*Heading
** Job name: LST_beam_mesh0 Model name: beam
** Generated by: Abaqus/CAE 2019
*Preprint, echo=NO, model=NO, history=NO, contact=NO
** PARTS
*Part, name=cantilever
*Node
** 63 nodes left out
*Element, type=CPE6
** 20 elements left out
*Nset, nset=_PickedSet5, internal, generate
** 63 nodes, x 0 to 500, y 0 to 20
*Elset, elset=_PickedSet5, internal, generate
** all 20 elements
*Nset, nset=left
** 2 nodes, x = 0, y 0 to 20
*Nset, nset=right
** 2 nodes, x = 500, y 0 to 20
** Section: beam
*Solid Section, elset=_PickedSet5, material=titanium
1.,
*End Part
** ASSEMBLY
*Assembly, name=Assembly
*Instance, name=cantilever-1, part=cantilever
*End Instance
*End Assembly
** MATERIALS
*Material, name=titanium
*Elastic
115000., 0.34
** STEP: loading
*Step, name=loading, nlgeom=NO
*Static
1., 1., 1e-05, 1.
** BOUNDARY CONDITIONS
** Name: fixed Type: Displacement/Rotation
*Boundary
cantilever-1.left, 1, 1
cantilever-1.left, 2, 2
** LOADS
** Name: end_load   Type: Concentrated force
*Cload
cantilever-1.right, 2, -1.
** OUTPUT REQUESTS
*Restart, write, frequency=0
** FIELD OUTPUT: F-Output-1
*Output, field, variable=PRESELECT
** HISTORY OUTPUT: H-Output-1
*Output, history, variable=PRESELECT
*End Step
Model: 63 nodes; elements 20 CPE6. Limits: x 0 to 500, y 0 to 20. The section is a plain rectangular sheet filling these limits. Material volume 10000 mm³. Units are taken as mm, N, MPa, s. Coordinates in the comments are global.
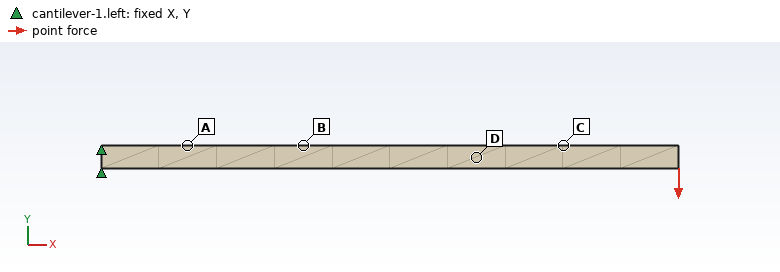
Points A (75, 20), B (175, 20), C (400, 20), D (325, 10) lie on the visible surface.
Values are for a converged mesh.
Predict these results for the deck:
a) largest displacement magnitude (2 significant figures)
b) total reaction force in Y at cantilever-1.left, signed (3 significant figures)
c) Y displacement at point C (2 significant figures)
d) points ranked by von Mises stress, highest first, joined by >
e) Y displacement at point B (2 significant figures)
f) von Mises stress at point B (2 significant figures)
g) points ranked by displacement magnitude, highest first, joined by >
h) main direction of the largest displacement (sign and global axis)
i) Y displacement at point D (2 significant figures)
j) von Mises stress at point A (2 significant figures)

0.98 mm
2.00 N
-0.69 mm
A > B > C > D
-0.16 mm
8.6 MPa
C > D > B > A
-Y
-0.49 mm
11 MPa
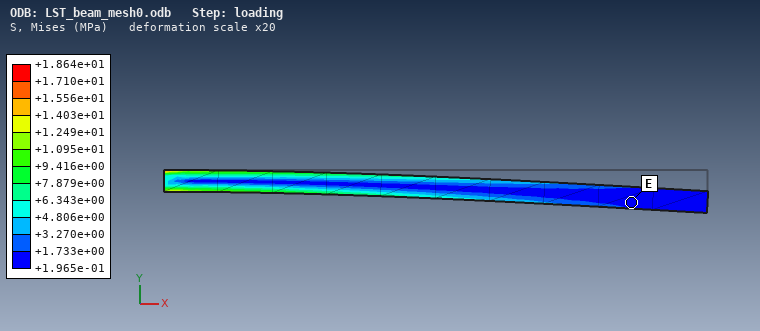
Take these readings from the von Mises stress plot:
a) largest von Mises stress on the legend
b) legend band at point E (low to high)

+1.864e+01 MPa
+1.965e-01 to +1.733e+00 MPa
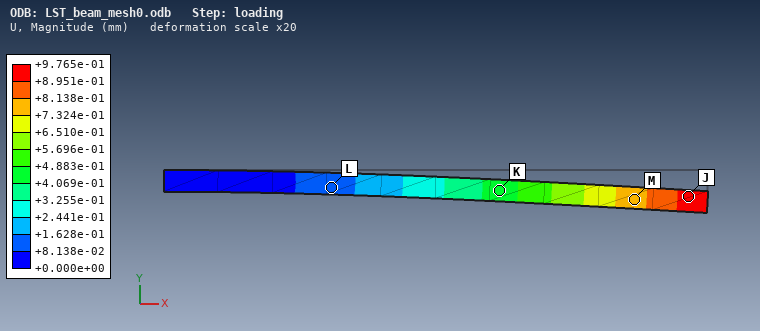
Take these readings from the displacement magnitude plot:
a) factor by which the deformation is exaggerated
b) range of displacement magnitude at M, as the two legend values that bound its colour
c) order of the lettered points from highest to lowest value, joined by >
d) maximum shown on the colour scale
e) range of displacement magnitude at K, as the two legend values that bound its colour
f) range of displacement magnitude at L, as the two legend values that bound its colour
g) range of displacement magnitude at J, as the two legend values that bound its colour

20
+7.324e-01 to +8.138e-01 mm
J > M > K > L
+9.765e-01 mm
+4.069e-01 to +4.883e-01 mm
+8.138e-02 to +1.628e-01 mm
+8.951e-01 to +9.765e-01 mm
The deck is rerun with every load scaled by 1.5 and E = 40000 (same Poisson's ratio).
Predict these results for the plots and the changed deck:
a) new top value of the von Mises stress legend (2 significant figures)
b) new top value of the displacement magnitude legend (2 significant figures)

28 MPa
4.2 mm
